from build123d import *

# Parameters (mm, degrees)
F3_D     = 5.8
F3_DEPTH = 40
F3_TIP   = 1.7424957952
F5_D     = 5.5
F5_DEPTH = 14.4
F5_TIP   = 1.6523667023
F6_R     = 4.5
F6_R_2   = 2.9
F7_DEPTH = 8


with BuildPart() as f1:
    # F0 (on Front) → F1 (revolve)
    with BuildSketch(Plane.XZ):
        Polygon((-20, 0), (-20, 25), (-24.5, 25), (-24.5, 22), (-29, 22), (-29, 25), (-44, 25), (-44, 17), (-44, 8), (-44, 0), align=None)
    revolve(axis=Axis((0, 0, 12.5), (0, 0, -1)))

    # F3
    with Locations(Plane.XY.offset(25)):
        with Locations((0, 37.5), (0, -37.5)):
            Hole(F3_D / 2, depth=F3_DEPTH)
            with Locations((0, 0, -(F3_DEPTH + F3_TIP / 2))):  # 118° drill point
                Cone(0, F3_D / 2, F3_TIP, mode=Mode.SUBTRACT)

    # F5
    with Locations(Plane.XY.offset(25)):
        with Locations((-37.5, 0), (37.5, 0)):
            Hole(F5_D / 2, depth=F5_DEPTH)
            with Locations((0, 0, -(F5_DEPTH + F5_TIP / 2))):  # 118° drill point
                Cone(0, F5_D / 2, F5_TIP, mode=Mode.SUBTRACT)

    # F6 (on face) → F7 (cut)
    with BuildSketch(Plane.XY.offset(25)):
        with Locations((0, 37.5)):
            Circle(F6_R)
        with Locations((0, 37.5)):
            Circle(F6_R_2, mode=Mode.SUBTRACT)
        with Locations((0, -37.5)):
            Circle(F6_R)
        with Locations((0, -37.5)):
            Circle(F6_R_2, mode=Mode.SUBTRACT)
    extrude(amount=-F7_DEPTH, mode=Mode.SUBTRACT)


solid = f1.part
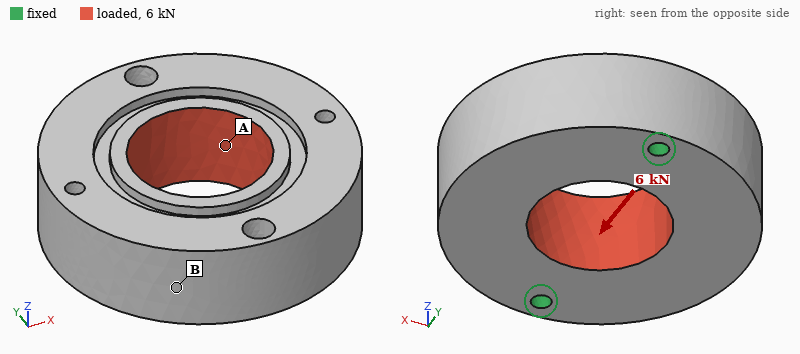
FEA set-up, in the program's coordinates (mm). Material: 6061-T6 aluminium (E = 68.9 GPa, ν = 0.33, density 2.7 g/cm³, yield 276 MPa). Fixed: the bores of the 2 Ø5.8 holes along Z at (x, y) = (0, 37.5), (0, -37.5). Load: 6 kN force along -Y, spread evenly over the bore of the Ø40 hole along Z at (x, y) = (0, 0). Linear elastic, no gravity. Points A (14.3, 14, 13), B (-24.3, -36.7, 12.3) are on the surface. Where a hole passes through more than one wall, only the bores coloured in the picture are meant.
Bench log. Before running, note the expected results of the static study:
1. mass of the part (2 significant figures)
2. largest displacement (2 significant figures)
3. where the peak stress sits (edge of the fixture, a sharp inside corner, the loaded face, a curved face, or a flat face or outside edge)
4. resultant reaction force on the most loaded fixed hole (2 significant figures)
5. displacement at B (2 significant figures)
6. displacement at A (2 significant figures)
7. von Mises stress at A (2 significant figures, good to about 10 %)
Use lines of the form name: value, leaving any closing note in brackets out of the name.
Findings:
mass of the part: 310 g
largest displacement: 3.9 µm
where the peak stress sits: edge of the fixture
resultant reaction force on the most loaded fixed hole: 3.0 kN
displacement at B: 2.9 µm
displacement at A: 3.1 µm
von Mises stress at A: 5.9 MPa
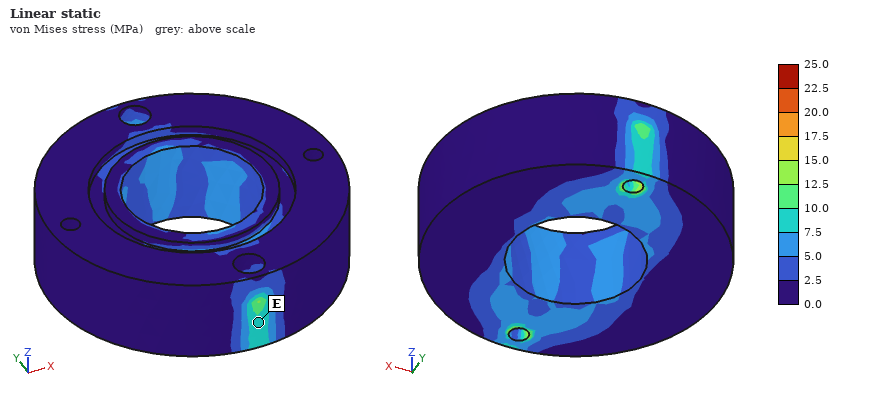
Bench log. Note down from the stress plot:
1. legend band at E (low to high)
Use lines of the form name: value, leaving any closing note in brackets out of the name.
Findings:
legend band at E: 7.5 to 10.0 MPa
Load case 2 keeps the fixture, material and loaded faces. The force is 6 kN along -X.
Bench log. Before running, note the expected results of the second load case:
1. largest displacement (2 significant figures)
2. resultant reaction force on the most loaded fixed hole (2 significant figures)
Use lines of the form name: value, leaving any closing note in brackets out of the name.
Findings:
largest displacement: 7.0 µm
resultant reaction force on the most loaded fixed hole: 3.0 kN
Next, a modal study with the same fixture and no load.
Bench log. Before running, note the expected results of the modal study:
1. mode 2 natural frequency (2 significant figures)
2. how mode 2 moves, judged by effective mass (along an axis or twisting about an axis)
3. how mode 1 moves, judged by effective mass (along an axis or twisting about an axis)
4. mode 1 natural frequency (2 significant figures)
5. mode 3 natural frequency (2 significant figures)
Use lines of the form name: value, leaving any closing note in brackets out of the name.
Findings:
mode 2 natural frequency: 6500 Hz
how mode 2 moves, judged by effective mass: along Z
how mode 1 moves, judged by effective mass: twisting about Y
mode 1 natural frequency: 4500 Hz
mode 3 natural frequency: 11 kHz
